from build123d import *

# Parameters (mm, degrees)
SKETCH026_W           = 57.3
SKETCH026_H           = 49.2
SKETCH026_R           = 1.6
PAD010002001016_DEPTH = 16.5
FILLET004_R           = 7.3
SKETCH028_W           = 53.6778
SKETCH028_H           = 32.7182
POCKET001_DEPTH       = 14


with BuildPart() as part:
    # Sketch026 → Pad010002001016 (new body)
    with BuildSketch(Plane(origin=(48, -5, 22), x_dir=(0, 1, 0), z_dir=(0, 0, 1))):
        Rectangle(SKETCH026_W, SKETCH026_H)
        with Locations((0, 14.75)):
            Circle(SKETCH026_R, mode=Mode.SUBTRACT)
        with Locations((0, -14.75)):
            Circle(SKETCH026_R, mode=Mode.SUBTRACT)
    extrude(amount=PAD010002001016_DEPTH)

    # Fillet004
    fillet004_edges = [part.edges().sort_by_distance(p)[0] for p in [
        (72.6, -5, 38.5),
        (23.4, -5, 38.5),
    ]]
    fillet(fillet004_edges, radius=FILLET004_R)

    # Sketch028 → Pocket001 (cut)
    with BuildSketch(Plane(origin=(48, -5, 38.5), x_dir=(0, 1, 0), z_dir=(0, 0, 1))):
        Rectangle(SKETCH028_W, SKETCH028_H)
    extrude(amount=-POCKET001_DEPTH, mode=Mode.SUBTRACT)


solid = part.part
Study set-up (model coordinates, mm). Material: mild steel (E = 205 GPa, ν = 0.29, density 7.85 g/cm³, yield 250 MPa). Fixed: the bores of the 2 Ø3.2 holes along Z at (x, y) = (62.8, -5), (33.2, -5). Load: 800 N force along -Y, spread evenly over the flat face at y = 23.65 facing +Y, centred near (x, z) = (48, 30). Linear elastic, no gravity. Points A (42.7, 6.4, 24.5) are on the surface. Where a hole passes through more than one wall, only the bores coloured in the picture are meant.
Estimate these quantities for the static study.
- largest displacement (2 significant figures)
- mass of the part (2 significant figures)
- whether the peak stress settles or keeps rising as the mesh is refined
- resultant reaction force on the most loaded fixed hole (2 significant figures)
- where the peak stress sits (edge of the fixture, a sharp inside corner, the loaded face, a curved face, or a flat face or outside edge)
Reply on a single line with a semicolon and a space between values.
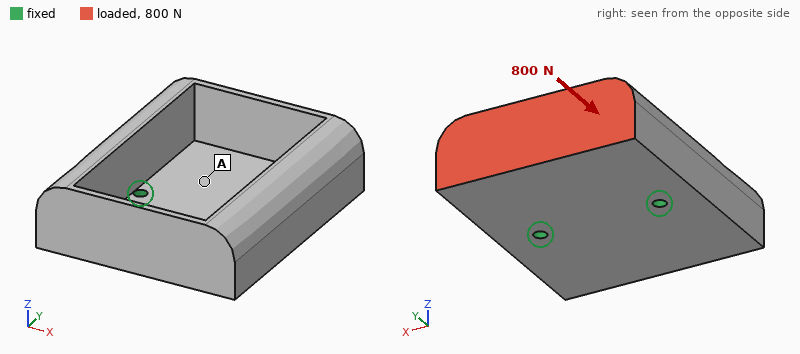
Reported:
45 µm; 160 g; keeps rising; 400 N; edge of the fixture
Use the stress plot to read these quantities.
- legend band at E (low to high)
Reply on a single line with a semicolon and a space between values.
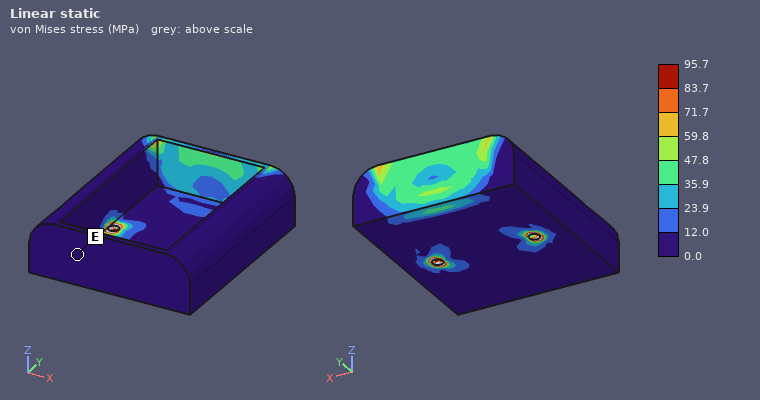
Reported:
0.0 to 12.0 MPa
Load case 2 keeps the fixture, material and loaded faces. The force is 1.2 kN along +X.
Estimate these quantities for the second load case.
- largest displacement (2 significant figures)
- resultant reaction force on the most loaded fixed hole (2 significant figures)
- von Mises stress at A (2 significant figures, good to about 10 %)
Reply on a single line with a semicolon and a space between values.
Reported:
20 µm; 1.3 kN; 33 MPa
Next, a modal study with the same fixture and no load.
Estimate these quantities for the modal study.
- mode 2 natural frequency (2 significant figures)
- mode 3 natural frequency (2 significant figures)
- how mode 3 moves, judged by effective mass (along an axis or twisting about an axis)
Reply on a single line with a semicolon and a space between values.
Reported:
4600 Hz; 5600 Hz; along X
